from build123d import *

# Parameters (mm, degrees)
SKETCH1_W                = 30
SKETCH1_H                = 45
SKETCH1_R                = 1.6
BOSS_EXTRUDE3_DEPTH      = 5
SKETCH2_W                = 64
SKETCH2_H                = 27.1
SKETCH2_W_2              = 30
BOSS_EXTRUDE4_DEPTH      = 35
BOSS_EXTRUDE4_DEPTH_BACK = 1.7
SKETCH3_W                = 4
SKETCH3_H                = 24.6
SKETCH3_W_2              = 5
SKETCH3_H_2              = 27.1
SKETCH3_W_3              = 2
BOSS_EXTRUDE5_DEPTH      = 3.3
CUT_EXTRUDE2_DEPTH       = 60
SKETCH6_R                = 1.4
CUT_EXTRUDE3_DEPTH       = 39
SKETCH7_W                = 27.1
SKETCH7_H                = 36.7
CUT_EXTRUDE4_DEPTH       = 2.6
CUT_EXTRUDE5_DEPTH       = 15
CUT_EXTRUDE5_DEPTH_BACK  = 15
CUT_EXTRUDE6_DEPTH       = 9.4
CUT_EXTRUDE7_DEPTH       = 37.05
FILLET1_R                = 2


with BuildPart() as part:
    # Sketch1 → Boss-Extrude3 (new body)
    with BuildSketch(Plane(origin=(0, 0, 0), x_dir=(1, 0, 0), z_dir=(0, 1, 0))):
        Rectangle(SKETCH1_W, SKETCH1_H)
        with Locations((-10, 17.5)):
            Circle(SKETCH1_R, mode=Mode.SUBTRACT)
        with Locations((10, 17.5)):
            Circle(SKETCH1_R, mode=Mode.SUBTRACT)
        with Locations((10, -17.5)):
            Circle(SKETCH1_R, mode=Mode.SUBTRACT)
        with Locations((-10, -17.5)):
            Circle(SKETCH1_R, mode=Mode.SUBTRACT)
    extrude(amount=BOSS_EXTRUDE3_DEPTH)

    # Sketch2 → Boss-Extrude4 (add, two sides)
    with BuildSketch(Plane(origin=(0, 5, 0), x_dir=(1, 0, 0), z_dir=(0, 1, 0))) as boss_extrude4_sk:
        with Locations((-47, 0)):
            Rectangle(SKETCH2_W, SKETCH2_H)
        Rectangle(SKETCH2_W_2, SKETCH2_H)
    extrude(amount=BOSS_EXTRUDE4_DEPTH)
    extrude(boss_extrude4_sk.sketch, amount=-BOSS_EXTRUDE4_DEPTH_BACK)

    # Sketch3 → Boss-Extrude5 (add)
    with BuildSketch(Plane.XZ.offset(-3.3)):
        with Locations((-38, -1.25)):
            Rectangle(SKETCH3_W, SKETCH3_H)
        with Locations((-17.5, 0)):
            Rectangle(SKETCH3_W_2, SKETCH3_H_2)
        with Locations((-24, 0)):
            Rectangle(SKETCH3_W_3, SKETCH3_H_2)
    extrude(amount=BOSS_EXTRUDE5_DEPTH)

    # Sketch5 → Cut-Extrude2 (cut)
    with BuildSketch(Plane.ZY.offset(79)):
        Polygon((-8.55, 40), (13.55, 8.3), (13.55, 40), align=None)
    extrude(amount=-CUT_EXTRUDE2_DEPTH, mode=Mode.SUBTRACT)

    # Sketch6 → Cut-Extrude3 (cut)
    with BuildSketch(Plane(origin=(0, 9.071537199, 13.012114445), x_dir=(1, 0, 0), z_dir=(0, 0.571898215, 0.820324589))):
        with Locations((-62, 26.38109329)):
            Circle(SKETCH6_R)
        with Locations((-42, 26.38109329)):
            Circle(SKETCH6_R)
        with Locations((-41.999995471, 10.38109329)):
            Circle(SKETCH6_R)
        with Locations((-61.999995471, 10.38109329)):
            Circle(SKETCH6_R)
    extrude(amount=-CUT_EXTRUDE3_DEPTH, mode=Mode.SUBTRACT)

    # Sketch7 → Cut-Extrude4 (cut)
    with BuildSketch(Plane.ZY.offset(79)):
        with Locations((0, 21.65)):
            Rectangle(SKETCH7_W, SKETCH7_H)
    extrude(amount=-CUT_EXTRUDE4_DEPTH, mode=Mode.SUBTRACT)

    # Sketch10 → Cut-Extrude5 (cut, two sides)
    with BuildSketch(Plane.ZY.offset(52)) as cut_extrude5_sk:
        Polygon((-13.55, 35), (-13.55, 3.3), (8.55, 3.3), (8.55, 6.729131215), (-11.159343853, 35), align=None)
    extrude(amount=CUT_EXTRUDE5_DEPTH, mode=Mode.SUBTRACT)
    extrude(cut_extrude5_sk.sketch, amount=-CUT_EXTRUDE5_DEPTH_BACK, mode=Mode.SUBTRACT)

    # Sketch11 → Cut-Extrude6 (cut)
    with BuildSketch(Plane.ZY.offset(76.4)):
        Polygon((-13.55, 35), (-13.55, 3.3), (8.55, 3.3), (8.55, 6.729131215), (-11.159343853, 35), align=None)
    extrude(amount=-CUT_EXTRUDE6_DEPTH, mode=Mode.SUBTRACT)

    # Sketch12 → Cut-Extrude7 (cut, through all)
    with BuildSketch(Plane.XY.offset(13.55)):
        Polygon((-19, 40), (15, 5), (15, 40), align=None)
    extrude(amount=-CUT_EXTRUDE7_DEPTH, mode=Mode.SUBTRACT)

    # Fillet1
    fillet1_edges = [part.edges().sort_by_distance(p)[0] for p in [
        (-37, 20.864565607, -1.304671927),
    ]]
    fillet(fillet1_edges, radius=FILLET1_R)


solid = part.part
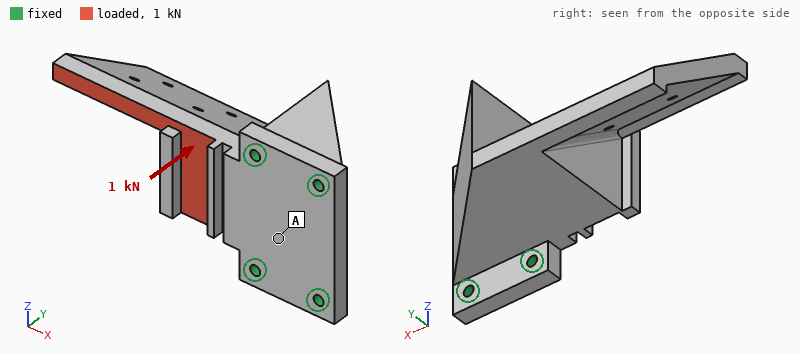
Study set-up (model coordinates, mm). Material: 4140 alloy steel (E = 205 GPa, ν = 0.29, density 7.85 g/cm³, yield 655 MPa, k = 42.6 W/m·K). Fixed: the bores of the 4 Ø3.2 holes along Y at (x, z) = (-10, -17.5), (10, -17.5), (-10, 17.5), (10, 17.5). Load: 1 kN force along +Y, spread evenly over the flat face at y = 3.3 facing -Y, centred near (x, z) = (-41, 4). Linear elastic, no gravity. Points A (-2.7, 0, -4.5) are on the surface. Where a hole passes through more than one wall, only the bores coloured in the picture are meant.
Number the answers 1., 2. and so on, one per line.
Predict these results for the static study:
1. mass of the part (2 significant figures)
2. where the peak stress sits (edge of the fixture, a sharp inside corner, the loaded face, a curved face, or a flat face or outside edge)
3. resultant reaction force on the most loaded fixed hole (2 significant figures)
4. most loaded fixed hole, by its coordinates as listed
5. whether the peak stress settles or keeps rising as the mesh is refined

1. 350 g
2. edge of the fixture
3. 1.4 kN
4. (-10, 17.5)
5. keeps rising
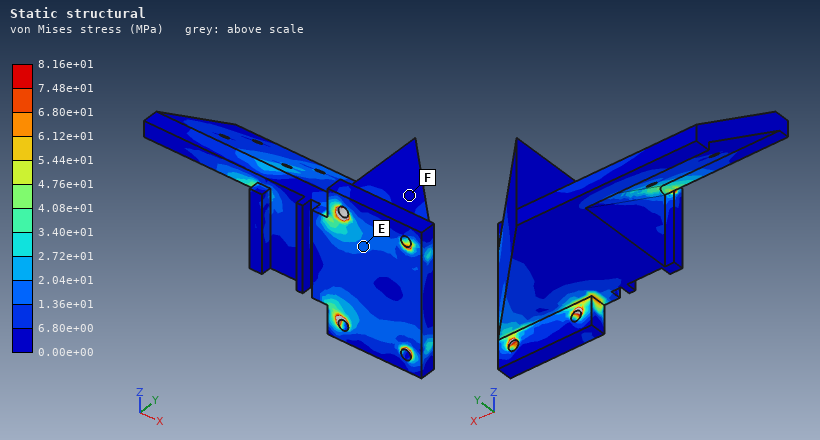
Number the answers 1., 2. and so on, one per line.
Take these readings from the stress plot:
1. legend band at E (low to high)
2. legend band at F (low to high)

1. 1.36e+01 to 2.04e+01 MPa
2. 0.00e+00 to 6.80e+00 MPa
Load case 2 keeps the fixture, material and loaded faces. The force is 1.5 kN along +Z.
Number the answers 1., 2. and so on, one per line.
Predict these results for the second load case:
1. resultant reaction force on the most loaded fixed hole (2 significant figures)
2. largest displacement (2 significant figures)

1. 1.2 kN
2. 89 µm
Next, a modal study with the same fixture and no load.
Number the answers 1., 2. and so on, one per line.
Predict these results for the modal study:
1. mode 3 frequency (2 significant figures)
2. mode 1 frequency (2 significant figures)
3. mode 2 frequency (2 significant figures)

1. 5000 Hz
2. 2100 Hz
3. 3100 Hz
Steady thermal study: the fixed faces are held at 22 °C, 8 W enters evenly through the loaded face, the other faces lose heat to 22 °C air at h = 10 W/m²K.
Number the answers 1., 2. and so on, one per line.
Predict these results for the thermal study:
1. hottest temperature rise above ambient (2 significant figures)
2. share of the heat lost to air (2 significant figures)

1. 23 K
2. 15 %
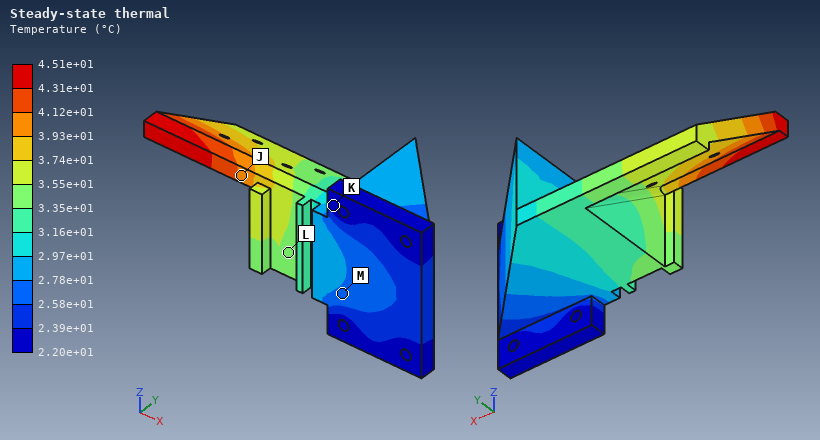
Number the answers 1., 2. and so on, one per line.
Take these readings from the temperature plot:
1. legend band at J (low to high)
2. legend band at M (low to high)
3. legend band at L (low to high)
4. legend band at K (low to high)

1. 3.93e+01 to 4.12e+01 °C
2. 2.58e+01 to 2.78e+01 °C
3. 3.35e+01 to 3.55e+01 °C
4. 2.20e+01 to 2.39e+01 °C
